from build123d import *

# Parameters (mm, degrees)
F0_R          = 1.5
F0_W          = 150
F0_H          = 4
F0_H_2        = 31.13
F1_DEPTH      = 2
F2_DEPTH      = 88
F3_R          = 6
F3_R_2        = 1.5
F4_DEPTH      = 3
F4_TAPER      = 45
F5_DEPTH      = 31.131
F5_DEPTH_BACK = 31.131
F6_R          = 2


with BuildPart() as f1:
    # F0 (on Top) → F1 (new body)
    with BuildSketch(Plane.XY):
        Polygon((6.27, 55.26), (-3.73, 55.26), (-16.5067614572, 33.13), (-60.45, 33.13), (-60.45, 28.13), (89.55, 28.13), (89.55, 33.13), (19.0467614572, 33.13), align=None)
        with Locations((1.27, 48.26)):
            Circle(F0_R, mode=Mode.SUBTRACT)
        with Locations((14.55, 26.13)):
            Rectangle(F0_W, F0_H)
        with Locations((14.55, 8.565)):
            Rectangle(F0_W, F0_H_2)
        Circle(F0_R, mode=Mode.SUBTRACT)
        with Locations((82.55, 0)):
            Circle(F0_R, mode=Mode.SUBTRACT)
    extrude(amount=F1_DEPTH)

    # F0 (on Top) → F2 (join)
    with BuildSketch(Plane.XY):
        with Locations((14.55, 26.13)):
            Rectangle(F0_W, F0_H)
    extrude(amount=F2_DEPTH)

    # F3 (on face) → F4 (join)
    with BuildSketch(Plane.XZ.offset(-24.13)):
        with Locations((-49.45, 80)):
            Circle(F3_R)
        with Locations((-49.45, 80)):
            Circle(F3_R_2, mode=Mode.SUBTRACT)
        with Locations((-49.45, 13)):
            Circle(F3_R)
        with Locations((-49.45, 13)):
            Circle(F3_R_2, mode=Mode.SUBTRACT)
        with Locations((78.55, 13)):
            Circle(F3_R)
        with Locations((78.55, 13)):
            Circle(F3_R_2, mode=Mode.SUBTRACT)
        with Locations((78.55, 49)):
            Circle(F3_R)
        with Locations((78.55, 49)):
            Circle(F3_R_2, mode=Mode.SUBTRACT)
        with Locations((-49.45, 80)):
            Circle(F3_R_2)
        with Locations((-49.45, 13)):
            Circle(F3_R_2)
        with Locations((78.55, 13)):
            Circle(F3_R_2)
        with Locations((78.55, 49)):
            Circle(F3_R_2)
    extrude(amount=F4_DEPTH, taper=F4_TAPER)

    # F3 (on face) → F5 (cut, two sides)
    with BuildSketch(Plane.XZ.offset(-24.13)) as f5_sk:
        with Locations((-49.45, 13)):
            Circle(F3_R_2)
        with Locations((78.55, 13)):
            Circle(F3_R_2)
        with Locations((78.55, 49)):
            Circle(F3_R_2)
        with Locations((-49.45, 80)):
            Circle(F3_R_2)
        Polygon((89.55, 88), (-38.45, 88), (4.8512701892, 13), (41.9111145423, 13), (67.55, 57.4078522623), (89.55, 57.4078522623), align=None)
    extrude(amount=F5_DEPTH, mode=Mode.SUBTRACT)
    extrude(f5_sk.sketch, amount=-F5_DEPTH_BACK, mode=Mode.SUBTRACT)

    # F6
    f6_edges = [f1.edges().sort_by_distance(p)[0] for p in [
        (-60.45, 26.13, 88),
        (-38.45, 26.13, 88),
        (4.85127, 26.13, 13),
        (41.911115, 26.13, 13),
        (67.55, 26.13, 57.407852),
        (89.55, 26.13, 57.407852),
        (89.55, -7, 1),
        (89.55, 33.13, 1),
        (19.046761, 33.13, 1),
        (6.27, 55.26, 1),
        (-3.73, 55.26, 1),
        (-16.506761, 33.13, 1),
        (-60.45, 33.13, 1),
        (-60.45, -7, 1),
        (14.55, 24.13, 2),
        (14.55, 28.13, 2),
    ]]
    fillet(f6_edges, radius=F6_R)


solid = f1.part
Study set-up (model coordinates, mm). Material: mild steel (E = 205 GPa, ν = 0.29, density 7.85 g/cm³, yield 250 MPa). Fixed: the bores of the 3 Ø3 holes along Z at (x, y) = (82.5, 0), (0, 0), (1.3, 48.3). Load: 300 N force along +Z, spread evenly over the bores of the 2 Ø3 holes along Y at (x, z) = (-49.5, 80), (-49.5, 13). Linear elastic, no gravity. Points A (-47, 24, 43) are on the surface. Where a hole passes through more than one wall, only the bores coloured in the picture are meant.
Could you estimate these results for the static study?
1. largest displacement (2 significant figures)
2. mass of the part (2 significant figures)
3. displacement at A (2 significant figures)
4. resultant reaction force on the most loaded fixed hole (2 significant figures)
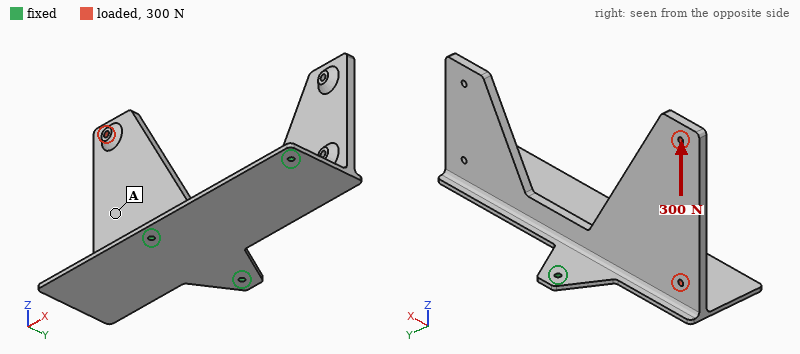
0.39 mm
310 g
0.25 mm
400 N
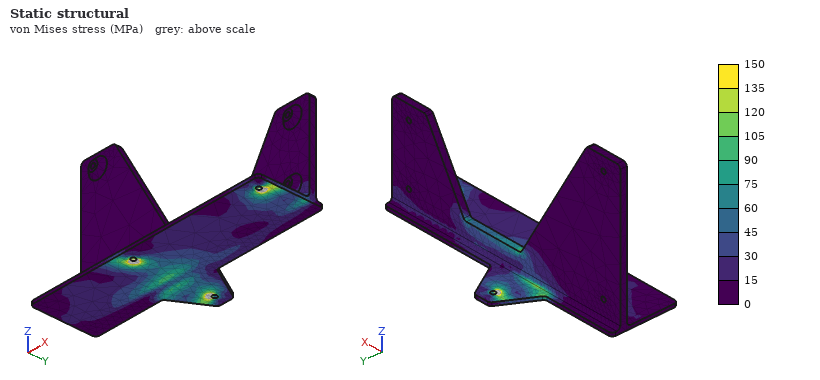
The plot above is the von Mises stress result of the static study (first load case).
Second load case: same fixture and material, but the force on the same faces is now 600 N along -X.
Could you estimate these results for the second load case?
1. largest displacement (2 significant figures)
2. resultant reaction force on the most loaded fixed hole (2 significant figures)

0.60 mm
720 N
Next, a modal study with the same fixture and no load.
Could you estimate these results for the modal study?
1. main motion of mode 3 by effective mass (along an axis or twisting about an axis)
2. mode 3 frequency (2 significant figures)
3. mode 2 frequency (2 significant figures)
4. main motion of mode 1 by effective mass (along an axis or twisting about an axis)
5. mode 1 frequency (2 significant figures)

along Z
620 Hz
370 Hz
along Y
320 Hz
